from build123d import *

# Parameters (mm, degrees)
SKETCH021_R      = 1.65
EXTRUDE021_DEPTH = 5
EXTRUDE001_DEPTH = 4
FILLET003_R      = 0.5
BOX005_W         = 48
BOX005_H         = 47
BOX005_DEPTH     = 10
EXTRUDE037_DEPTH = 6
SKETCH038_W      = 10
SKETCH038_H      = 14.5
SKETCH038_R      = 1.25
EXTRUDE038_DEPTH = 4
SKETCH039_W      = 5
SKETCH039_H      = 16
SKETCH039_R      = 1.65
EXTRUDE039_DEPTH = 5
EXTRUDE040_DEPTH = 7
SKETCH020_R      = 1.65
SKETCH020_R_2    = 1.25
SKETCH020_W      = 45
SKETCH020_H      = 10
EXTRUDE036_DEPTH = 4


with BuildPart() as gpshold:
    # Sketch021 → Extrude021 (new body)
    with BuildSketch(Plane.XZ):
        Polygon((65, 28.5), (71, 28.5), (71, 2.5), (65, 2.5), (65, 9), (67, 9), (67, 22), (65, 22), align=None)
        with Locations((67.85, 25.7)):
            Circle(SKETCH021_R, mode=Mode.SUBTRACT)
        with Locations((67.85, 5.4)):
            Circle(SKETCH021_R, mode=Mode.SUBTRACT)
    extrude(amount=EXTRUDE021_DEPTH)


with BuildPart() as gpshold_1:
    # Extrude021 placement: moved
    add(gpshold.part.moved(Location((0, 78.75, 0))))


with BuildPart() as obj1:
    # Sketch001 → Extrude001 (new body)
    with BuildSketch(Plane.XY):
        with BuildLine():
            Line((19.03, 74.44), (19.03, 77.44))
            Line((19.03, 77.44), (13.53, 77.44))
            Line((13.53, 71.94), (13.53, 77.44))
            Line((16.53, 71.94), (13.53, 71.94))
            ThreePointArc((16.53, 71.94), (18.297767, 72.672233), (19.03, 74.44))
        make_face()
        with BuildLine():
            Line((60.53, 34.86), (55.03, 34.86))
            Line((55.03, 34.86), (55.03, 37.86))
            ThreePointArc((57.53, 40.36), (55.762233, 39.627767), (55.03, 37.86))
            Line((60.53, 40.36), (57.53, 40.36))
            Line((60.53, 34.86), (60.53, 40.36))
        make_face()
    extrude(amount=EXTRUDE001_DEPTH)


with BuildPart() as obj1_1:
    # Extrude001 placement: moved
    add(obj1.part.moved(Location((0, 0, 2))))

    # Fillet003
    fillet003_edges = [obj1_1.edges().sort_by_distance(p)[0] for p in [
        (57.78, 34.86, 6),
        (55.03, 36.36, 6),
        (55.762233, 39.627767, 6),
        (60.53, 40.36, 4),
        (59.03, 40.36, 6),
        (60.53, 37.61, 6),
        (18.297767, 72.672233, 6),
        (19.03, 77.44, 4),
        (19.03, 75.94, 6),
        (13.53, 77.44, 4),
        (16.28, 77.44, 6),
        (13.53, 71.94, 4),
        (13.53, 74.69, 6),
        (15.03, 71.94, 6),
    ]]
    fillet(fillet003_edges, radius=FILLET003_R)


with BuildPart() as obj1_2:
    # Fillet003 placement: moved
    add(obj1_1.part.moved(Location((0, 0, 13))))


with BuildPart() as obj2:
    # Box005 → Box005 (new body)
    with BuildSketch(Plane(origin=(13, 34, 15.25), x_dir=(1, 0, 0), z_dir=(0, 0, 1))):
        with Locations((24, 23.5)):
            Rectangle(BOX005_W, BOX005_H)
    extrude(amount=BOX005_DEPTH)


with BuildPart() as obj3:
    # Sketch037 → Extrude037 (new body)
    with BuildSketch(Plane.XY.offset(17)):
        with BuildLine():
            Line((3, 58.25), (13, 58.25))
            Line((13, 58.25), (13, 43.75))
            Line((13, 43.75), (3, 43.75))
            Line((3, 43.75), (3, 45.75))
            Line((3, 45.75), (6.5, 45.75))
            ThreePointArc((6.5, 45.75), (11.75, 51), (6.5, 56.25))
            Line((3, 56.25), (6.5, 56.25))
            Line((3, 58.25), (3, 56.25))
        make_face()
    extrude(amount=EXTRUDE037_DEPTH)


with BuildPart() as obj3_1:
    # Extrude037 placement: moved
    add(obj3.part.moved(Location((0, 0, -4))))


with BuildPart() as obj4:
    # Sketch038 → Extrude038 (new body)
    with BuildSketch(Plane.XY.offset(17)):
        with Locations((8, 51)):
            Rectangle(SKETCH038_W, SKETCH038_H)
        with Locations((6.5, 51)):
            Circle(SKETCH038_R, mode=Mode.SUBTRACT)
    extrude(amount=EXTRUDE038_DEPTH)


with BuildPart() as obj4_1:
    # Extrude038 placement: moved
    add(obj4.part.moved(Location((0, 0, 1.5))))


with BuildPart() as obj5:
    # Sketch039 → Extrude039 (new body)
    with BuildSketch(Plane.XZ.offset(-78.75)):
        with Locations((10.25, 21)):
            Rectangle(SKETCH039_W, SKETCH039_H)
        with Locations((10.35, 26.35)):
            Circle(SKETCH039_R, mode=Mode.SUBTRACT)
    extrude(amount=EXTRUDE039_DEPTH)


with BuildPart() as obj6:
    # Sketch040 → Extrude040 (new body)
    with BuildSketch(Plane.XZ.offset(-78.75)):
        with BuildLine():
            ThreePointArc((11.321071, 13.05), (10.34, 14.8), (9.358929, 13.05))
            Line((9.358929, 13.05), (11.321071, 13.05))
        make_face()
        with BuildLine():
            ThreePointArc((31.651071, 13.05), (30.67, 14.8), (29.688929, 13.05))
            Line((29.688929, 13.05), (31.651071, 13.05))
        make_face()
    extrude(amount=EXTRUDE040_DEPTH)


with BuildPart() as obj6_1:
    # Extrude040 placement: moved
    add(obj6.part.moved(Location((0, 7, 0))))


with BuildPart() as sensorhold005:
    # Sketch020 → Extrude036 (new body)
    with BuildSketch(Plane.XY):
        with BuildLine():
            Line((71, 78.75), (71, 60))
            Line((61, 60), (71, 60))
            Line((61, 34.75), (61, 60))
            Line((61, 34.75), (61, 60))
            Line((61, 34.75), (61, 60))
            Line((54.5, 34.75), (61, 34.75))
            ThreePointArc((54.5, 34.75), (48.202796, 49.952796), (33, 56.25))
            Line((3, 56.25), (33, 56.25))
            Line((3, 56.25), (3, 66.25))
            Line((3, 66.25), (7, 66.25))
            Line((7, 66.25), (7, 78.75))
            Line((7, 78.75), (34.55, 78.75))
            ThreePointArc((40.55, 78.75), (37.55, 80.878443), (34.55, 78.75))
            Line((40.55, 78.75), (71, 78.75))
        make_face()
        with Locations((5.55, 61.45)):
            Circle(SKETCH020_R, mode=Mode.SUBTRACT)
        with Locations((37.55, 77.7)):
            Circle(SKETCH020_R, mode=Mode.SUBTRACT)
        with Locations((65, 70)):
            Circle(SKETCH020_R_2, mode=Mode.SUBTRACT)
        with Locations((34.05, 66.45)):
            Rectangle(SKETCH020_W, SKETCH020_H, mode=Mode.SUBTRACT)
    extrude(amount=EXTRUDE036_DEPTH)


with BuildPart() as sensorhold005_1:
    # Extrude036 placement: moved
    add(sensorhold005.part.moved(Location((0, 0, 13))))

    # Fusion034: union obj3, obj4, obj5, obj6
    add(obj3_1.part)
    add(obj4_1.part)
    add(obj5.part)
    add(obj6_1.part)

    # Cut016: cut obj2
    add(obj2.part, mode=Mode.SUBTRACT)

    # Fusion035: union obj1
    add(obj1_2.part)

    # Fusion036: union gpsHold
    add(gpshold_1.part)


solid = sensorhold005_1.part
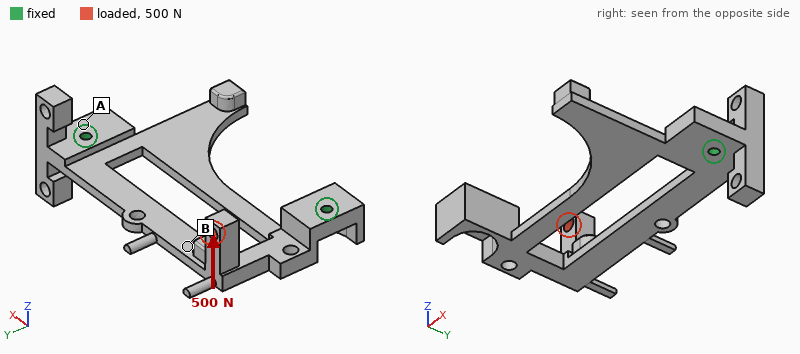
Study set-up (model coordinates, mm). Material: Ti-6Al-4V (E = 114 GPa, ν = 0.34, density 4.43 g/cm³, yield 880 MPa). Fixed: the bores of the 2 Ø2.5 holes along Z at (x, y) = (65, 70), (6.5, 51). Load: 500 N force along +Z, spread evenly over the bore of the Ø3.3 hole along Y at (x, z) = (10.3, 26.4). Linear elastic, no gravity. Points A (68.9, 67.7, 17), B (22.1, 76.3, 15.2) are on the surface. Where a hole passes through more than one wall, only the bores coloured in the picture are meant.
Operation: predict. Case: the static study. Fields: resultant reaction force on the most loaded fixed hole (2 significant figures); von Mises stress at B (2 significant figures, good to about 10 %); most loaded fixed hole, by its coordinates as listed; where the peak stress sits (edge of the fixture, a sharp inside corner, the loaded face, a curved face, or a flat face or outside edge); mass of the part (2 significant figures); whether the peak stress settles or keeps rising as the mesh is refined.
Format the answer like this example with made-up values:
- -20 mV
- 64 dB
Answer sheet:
- 530 N
- 140 MPa
- (6.5, 51)
- edge of the fixture
- 23 g
- keeps rising
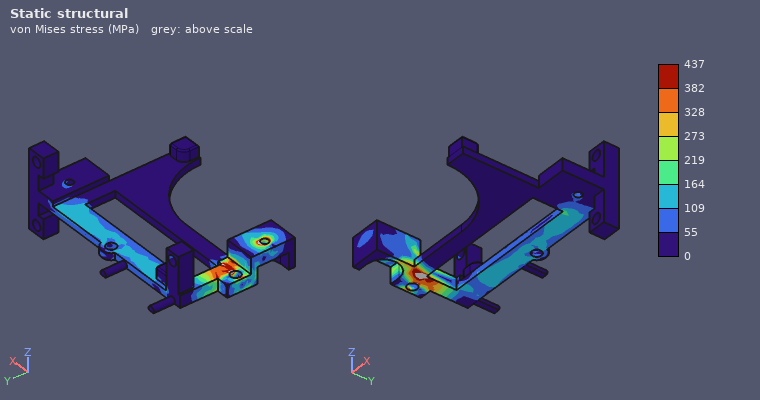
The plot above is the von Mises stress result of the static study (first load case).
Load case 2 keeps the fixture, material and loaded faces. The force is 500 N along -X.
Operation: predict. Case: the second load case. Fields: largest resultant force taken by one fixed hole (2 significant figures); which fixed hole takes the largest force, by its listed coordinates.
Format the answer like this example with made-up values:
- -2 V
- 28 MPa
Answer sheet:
- 360 N
- (65, 70)
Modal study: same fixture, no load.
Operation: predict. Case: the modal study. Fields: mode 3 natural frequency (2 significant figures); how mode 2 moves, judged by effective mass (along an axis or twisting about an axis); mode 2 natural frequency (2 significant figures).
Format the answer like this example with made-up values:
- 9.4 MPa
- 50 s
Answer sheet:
- 4000 Hz
- along Z
- 2300 Hz
